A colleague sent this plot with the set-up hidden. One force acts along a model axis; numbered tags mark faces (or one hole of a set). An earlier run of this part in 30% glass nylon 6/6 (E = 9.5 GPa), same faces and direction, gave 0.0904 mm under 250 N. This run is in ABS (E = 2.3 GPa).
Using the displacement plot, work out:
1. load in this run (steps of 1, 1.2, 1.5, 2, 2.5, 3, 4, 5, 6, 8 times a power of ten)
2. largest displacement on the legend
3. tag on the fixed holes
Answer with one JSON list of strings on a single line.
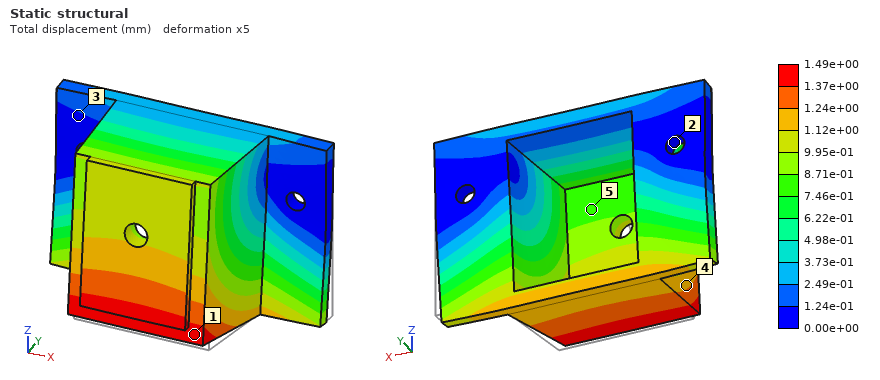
["1 kN", "1.49e+00 mm", "2"]
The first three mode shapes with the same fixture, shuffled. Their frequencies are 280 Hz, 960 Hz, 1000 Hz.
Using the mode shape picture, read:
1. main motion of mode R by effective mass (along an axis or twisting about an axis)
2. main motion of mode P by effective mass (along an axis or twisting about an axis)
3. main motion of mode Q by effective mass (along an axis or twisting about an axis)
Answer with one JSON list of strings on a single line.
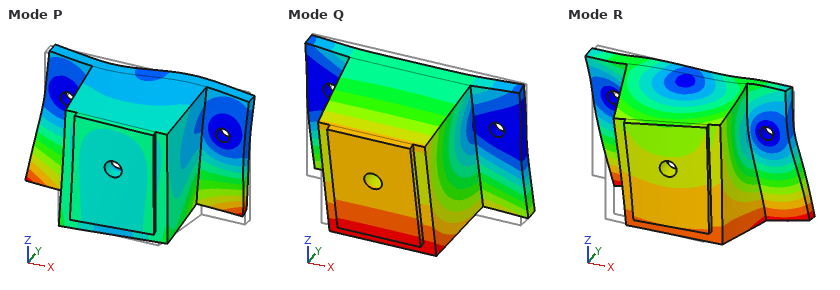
["along X", "twisting about Z", "along Z"]
